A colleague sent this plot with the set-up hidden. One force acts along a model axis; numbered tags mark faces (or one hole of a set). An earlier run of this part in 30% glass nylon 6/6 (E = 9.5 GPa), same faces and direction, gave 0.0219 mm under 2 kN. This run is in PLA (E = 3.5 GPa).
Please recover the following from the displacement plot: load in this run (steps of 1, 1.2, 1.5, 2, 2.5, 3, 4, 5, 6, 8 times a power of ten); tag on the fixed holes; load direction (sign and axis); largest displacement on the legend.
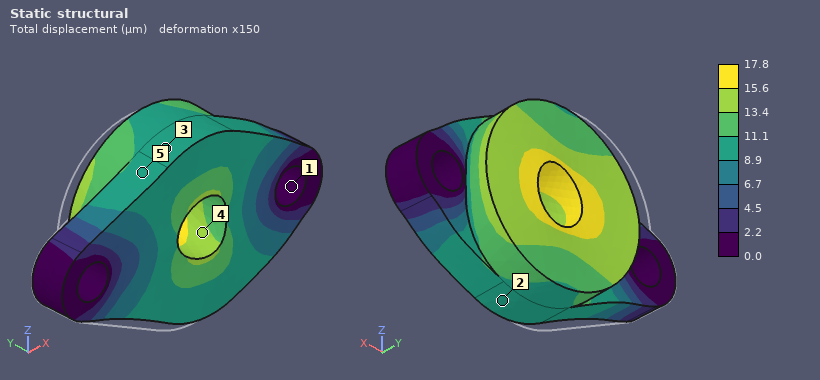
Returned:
600 N
1
+X
17.8 µm
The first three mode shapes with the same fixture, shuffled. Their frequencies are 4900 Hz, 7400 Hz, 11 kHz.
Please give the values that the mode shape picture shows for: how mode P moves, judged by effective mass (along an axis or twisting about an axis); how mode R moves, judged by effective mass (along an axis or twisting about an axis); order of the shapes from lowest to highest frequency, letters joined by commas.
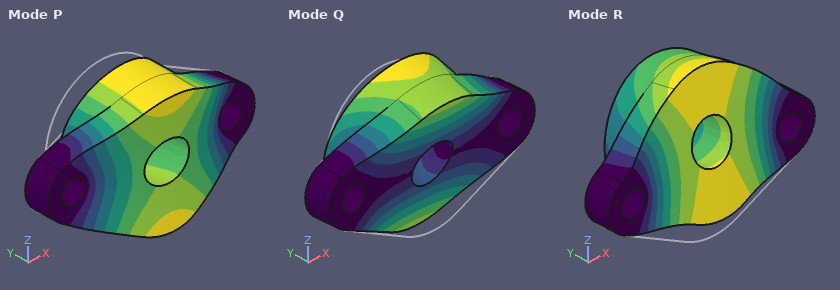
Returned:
along Y
along Z
Q, P, R
